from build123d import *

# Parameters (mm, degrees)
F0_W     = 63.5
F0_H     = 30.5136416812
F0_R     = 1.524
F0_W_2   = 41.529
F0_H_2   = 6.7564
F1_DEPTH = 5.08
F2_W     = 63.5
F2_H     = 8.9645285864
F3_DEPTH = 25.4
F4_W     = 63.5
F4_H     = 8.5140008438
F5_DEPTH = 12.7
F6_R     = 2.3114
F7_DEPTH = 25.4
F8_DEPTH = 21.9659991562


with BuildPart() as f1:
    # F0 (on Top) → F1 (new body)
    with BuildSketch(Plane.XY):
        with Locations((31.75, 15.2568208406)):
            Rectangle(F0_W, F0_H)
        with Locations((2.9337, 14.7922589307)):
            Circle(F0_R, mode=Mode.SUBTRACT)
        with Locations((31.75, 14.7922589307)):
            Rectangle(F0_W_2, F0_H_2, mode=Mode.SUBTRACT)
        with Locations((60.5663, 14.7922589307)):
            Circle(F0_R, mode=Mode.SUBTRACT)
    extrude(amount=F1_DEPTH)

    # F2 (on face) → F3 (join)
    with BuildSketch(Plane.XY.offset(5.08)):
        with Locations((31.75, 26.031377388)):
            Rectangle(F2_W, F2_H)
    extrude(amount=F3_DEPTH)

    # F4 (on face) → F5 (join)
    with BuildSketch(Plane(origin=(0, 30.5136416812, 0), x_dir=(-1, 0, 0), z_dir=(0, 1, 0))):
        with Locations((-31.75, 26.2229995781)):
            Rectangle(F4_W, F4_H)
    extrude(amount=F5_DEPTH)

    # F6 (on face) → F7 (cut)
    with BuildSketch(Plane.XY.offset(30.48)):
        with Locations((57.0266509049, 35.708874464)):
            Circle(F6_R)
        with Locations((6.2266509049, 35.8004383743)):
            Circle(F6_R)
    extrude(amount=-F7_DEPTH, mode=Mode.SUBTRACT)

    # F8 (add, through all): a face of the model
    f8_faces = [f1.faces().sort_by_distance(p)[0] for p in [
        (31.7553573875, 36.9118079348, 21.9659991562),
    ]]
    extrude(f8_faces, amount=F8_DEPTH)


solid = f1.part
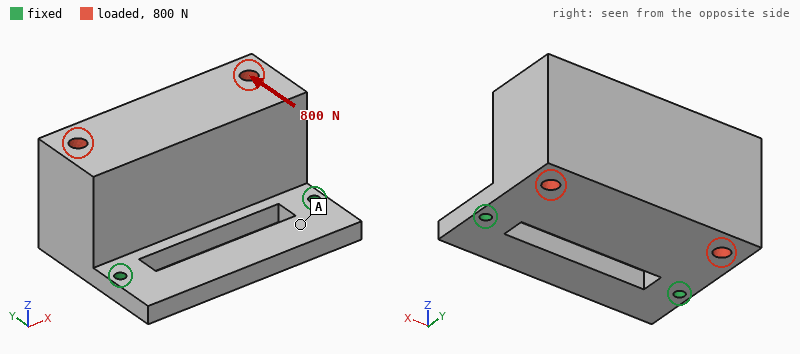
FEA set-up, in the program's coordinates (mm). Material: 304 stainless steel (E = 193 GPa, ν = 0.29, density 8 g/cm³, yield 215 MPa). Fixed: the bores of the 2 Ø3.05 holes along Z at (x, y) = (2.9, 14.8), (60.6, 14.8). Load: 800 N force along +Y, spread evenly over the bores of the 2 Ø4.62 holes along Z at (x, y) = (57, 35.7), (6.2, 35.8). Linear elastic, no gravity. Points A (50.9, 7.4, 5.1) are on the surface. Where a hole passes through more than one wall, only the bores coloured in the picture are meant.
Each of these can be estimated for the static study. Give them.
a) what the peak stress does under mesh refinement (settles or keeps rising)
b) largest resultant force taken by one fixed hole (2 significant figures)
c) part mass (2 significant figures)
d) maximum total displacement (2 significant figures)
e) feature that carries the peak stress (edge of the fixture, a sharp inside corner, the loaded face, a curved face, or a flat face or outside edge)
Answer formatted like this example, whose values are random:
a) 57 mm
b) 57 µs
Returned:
a) keeps rising
b) 400 N
c) 370 g
d) 71 µm
e) edge of the fixture
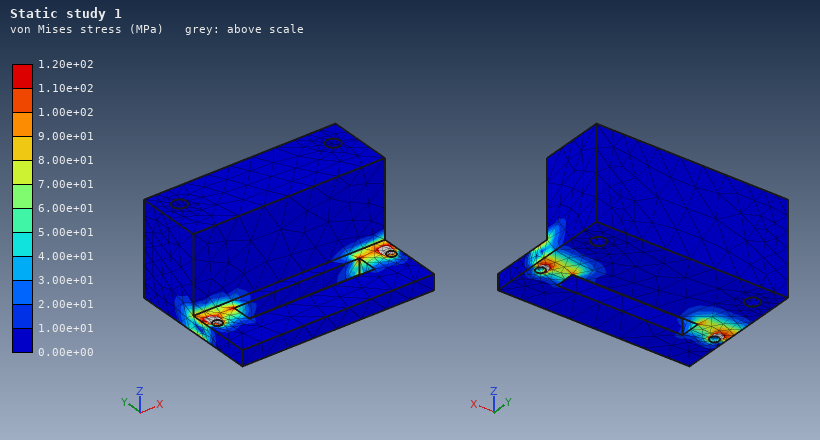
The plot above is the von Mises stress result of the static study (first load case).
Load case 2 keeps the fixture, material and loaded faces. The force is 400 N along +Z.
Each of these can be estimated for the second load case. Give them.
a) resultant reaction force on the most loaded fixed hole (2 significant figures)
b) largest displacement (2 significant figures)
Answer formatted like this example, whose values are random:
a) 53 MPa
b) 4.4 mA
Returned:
a) 200 N
b) 47 µm
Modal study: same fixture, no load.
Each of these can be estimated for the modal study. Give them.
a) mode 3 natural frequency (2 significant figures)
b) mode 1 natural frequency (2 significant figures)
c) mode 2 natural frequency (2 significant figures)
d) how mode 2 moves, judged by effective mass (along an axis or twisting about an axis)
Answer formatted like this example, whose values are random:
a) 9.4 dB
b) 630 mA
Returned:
a) 5900 Hz
b) 950 Hz
c) 5100 Hz
d) along X
